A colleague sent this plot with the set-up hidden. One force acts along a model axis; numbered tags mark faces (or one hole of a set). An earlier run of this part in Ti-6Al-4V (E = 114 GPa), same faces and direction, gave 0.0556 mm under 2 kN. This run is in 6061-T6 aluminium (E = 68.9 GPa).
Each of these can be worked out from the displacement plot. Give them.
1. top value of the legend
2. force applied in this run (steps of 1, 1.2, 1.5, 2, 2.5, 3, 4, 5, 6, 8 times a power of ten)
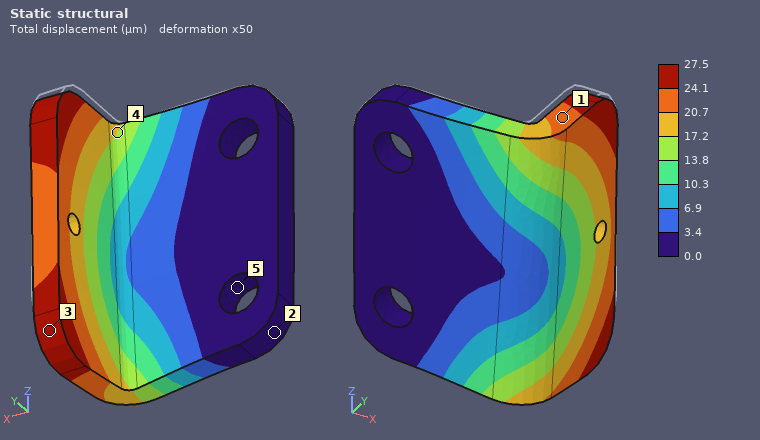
27.5 µm
600 N
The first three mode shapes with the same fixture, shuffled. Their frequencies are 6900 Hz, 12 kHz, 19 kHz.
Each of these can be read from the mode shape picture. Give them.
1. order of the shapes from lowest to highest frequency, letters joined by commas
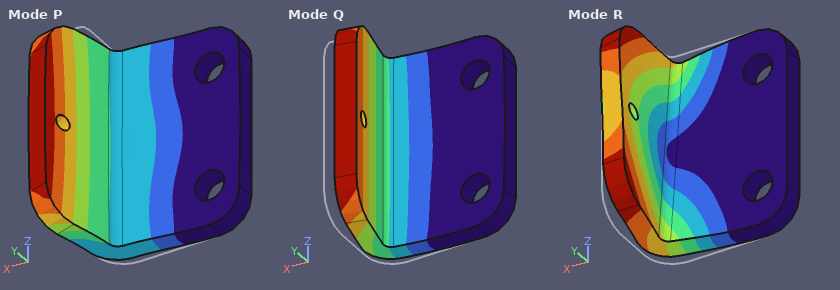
Q, R, P
